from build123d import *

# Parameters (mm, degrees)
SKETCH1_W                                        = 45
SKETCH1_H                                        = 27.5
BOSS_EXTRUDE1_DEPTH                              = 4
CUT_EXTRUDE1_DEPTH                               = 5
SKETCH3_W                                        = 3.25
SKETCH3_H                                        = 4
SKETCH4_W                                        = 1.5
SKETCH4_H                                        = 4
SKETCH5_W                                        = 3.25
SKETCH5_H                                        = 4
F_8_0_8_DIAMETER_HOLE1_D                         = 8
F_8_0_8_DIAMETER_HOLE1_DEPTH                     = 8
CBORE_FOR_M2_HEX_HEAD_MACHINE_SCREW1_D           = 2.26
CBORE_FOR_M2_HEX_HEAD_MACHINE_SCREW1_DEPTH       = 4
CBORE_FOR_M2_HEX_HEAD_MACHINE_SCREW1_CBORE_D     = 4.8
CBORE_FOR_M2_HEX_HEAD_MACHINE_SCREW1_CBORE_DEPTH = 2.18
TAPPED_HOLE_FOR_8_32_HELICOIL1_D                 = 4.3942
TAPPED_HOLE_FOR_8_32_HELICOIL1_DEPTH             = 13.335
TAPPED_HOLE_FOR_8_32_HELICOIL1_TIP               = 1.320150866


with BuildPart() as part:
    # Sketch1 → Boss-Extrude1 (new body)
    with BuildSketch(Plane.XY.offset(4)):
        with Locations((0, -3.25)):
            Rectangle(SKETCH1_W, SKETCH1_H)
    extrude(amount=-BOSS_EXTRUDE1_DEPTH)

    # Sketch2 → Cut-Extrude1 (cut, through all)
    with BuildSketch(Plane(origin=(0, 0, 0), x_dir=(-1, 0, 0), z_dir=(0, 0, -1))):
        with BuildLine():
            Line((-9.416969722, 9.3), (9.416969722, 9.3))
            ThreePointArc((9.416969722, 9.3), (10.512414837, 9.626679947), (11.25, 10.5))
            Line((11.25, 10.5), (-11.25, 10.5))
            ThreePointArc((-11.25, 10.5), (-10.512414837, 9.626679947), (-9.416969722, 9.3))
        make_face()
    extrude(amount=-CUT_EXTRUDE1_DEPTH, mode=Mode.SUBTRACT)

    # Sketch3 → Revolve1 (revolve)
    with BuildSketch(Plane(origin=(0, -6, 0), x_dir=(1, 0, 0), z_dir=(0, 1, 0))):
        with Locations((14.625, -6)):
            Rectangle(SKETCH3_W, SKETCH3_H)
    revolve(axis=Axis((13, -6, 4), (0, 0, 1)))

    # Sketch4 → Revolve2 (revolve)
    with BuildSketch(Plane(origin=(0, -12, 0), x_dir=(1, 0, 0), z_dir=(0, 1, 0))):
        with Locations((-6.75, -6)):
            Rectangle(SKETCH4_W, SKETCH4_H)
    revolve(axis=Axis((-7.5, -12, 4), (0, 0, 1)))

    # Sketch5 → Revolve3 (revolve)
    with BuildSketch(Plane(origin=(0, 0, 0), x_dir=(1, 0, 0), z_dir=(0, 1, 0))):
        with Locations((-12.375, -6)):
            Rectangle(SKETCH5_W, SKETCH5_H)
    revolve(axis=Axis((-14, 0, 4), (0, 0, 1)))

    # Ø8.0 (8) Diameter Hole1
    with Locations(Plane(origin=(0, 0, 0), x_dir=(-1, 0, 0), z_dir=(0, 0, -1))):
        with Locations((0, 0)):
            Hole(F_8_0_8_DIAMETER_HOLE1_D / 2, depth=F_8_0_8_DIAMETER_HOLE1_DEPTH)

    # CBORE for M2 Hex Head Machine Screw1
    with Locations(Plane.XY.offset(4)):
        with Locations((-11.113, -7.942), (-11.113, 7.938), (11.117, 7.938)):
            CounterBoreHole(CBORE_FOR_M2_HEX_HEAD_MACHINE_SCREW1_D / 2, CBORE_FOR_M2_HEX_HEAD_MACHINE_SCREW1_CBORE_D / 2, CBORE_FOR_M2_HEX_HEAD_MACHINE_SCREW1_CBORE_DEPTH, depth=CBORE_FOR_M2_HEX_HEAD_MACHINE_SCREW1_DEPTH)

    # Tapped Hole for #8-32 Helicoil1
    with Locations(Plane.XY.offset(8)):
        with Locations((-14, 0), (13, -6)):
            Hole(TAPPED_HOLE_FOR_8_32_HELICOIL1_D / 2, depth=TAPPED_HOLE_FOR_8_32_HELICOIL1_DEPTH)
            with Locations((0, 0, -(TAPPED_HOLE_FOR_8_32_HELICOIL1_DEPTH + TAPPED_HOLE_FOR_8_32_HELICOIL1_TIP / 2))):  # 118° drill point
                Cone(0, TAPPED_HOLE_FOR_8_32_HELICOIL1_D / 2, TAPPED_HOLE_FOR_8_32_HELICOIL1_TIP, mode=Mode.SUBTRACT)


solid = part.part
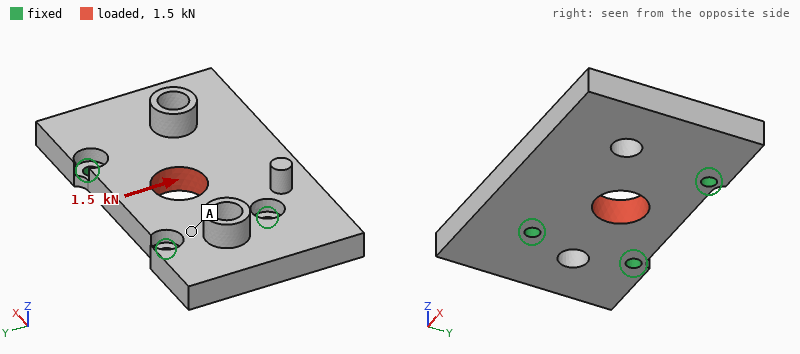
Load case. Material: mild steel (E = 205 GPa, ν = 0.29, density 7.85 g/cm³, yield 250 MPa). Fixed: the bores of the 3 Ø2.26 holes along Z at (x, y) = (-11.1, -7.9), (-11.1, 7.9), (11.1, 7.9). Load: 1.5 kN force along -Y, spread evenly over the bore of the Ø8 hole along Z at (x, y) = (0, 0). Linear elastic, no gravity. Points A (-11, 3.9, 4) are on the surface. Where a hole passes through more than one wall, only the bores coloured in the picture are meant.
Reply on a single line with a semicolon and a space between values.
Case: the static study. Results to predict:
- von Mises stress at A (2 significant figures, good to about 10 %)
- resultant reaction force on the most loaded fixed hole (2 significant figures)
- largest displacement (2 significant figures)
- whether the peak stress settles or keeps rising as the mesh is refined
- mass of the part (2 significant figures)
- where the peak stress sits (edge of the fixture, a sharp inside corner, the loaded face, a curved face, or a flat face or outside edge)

12 MPa; 620 N; 6.9 µm; keeps rising; 36 g; edge of the fixture
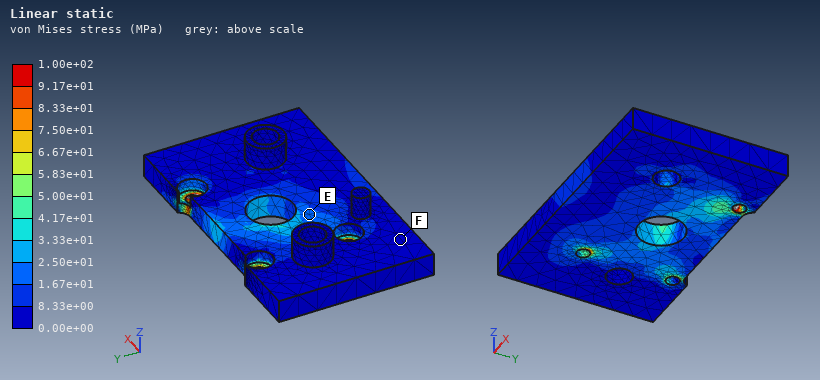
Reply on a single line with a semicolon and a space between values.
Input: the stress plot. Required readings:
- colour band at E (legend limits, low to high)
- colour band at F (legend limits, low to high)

1.67e+01 to 2.50e+01 MPa; 0.00e+00 to 8.33e+00 MPa
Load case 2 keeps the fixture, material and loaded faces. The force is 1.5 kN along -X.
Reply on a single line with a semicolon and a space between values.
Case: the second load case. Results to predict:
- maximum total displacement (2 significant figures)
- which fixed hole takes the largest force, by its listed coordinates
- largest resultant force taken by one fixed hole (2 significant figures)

4.7 µm; (-11.1, -7.9); 620 N
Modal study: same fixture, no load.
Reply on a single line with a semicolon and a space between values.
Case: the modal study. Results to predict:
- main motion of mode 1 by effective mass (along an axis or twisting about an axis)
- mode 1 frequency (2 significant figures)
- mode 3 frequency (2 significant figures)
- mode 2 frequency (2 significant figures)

along Z; 4500 Hz; 15 kHz; 12 kHz
